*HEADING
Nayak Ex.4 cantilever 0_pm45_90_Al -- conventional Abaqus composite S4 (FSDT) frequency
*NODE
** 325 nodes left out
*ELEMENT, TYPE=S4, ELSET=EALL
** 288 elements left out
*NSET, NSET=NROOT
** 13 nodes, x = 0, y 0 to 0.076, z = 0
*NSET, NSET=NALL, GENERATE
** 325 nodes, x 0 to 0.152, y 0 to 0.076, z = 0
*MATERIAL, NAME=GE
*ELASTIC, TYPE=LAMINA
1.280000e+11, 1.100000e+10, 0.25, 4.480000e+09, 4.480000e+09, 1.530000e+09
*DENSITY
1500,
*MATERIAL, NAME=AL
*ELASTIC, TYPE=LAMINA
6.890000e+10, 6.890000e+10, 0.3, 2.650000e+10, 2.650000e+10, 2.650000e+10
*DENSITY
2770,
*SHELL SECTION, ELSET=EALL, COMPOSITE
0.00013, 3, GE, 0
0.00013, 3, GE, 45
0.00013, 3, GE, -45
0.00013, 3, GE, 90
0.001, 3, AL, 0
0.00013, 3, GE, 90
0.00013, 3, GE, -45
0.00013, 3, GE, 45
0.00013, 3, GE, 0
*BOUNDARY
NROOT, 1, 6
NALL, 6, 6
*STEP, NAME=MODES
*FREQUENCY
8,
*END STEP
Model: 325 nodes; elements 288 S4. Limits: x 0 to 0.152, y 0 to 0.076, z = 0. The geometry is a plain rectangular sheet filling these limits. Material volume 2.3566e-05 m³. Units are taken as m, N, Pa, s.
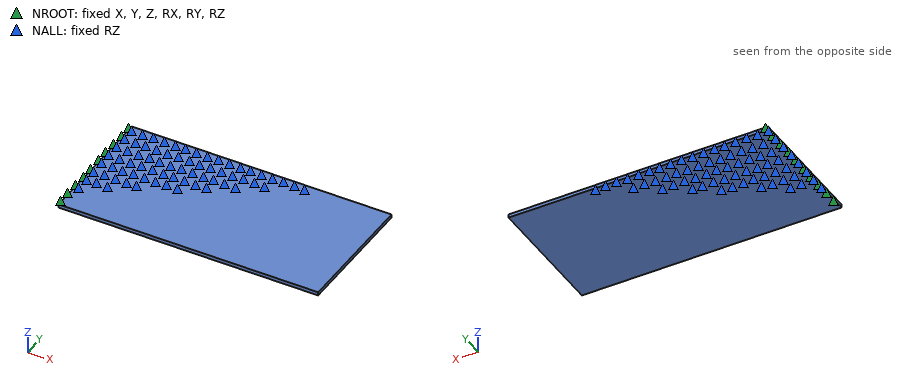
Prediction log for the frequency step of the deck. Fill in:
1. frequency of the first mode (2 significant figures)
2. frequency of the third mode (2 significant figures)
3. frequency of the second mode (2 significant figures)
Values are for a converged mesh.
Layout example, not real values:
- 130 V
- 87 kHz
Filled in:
- 81 Hz
- 500 Hz
- 310 Hz
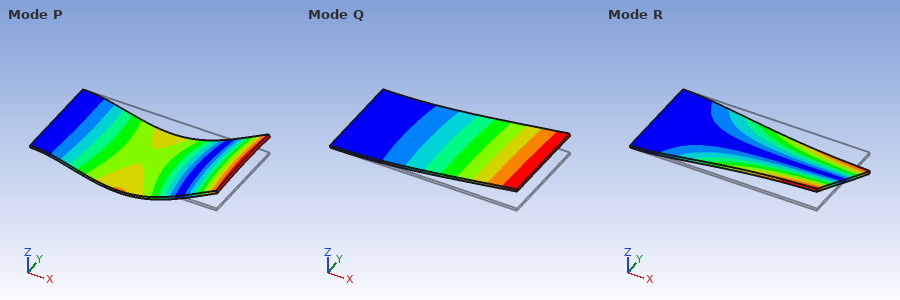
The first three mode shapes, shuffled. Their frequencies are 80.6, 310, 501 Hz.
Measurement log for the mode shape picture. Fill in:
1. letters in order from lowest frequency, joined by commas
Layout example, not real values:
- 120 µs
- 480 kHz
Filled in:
- Q, R, P
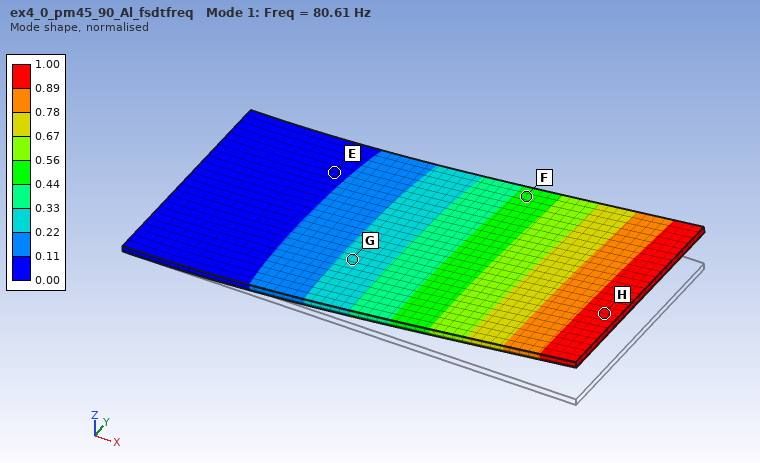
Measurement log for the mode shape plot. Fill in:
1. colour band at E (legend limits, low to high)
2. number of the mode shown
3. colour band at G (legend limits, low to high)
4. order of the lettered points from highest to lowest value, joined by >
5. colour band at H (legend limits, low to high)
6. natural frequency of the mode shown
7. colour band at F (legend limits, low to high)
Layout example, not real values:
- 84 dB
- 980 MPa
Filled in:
- 0.00 to 0.11
- 1
- 0.22 to 0.33
- H > F > G > E
- 0.89 to 1.00
- 80.61 Hz
- 0.44 to 0.56
